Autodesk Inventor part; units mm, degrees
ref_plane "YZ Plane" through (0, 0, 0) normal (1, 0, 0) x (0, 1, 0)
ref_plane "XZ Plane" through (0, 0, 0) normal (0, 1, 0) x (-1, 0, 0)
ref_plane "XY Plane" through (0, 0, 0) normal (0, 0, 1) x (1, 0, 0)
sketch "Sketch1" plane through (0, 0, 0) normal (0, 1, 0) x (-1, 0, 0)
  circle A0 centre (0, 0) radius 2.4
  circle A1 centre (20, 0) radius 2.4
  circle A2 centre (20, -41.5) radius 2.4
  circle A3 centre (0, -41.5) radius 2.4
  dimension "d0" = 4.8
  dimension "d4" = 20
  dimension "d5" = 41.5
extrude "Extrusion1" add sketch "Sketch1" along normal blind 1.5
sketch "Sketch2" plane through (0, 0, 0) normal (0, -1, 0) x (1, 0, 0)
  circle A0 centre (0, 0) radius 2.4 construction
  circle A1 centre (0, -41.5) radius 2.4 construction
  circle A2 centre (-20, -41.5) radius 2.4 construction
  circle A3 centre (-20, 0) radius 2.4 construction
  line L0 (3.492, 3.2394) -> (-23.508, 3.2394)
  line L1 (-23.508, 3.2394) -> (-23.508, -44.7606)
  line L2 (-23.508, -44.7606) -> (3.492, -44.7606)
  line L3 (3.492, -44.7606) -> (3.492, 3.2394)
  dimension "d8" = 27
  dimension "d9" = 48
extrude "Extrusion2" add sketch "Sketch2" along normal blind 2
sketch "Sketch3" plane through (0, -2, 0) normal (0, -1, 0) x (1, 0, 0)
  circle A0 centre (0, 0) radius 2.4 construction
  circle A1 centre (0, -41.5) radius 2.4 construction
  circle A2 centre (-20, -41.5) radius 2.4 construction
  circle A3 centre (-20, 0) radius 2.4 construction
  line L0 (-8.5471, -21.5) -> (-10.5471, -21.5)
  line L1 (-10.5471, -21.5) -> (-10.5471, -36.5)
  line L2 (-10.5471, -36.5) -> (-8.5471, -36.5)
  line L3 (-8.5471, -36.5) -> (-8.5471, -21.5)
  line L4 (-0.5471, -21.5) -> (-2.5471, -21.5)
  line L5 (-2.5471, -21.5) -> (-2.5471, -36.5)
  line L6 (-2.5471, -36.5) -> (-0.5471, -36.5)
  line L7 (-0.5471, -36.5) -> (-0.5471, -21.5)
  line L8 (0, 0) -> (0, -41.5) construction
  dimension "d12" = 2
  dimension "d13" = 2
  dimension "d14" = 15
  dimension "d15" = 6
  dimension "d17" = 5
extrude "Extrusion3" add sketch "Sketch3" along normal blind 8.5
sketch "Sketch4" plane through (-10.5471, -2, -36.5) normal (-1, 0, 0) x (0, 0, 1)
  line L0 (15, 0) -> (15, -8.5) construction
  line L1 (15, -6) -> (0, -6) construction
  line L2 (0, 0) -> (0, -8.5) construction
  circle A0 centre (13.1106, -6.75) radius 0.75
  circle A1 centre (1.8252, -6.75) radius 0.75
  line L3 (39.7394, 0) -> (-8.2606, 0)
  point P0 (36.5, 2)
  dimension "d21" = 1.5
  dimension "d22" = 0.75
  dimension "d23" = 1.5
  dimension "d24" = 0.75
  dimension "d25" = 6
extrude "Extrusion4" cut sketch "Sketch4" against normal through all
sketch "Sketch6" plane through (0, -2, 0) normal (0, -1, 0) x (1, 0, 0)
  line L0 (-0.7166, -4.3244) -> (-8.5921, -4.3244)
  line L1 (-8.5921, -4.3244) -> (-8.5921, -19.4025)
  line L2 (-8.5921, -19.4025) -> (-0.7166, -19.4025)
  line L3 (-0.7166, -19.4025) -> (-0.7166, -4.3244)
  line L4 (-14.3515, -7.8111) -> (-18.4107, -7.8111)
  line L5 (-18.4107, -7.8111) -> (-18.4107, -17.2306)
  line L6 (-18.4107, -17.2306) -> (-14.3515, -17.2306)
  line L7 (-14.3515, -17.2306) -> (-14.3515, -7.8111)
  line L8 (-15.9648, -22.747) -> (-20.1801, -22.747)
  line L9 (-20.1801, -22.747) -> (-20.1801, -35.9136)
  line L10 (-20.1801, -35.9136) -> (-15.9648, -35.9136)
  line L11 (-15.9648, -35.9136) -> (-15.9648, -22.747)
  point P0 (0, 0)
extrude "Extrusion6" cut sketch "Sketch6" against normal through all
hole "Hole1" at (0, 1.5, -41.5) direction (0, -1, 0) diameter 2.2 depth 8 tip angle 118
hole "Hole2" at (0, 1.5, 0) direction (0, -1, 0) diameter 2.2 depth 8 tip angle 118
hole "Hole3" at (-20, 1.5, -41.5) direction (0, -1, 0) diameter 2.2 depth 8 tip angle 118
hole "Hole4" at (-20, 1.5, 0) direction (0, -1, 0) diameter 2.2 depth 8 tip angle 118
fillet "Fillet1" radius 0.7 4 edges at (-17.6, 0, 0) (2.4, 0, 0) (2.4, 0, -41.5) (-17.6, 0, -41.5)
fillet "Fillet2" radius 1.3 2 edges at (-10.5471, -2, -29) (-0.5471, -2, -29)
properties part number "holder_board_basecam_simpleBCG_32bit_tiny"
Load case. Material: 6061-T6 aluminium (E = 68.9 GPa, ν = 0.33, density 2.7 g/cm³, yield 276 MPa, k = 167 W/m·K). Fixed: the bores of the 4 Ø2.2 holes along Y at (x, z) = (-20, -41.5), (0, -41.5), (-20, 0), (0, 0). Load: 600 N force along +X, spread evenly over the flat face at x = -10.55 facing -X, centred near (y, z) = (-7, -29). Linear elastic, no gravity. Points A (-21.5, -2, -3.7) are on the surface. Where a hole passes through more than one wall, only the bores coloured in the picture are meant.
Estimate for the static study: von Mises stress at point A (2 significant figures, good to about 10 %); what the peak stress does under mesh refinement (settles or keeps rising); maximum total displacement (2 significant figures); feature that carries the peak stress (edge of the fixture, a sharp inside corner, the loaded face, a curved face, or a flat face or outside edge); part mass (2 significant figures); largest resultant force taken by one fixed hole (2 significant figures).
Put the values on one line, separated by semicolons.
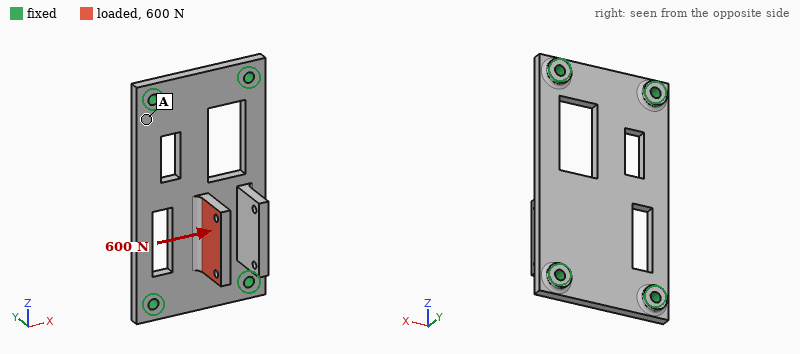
30 MPa; keeps rising; 0.18 mm; a sharp inside corner; 7.4 g; 410 N
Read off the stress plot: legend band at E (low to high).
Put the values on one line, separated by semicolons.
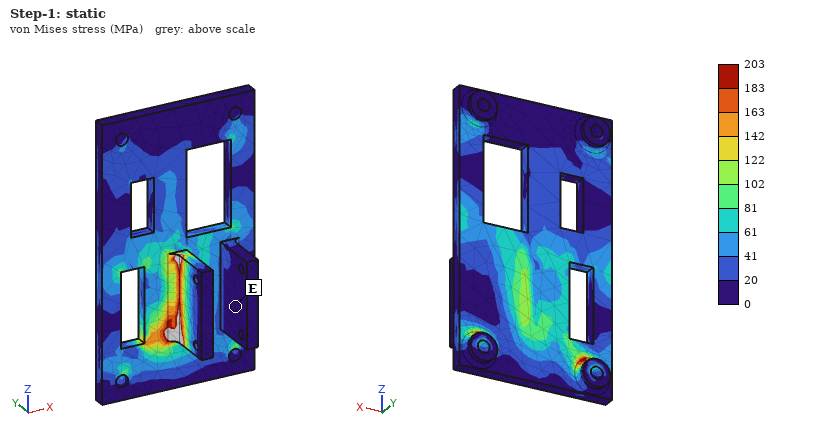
0 to 20 MPa
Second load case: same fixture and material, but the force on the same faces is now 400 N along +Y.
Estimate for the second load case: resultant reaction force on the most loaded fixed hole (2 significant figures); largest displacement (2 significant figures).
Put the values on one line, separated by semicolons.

170 N; 0.12 mm
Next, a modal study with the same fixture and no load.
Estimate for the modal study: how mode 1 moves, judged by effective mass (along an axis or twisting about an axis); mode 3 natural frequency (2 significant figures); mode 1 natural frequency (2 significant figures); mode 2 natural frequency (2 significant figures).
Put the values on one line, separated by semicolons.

along Y; 12 kHz; 5300 Hz; 8000 Hz
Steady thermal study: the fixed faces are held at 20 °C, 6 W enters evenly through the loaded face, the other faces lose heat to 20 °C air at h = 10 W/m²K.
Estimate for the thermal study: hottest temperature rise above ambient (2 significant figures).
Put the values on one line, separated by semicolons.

15 K
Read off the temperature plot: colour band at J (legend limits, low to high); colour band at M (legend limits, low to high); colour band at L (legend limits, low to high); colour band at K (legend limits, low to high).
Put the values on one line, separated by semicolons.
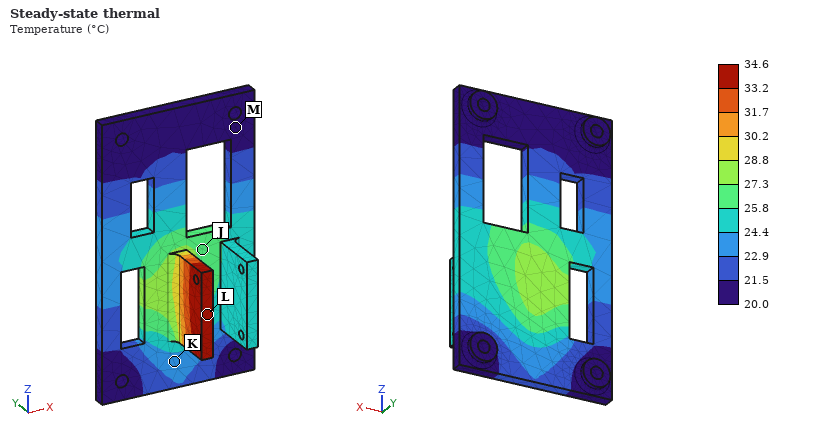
25.8 to 27.3 °C; 20.0 to 21.5 °C; 33.2 to 34.6 °C; 22.9 to 24.4 °C
